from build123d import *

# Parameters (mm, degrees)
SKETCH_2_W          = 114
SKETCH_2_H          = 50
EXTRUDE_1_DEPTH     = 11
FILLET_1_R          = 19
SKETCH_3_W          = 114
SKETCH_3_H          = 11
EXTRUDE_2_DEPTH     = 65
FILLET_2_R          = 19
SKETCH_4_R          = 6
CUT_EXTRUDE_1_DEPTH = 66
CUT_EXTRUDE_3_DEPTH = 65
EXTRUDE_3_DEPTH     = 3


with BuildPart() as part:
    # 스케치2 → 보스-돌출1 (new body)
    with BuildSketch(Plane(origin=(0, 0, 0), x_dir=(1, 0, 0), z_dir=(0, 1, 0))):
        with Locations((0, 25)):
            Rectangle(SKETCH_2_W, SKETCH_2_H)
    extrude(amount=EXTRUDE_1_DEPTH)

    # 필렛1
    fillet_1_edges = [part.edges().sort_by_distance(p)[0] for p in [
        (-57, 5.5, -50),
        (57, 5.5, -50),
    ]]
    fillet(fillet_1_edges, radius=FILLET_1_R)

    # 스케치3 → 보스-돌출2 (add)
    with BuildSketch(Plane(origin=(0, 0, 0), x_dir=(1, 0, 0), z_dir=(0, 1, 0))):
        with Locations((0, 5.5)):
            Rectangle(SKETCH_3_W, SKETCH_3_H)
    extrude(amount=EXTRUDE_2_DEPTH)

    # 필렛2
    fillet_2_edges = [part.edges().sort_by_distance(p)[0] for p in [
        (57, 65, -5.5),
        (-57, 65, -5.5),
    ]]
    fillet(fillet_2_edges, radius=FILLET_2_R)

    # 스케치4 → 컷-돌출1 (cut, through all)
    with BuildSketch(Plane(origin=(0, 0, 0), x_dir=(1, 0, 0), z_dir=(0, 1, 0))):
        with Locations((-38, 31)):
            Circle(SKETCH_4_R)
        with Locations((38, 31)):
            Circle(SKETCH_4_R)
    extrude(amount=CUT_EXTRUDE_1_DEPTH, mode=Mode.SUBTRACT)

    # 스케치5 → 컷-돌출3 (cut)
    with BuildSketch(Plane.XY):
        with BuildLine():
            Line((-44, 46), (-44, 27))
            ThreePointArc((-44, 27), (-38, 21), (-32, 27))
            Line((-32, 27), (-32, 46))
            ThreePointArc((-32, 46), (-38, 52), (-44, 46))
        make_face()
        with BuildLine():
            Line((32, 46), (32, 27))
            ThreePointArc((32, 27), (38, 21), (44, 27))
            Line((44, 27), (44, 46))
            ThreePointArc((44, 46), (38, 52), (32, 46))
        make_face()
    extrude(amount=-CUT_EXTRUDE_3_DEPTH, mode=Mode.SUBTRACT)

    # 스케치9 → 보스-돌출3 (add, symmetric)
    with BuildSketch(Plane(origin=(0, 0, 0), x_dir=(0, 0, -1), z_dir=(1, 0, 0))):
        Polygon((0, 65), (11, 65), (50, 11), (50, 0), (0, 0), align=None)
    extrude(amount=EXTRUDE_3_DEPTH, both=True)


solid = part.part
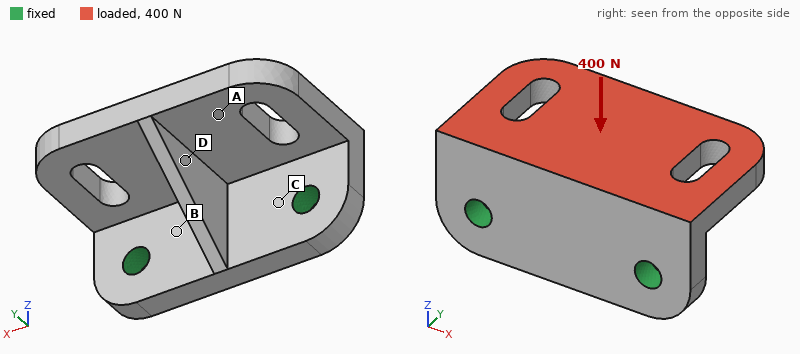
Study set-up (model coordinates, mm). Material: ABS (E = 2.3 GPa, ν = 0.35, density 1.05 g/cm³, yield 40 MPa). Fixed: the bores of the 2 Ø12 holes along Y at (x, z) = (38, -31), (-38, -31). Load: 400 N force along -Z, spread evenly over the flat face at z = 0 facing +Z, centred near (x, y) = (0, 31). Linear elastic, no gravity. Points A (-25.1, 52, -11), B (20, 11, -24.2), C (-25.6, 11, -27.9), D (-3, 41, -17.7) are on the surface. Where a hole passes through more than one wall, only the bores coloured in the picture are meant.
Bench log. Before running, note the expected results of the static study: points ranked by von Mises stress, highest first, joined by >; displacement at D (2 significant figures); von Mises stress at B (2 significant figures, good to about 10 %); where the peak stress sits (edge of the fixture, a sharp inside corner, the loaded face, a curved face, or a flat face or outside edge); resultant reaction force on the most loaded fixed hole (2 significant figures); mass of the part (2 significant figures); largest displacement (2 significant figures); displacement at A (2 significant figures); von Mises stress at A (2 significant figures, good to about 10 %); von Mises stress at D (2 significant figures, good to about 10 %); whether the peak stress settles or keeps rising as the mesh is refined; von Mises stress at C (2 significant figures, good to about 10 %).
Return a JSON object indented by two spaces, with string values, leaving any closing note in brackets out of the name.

{
  "points ranked by von Mises stress, highest first, joined by >": "C > B > D > A",
  "displacement at D": "0.23 mm",
  "von Mises stress at B": "2.4 MPa",
  "where the peak stress sits": "edge of the fixture",
  "resultant reaction force on the most loaded fixed hole": "200 N",
  "mass of the part": "130 g",
  "largest displacement": "0.46 mm",
  "displacement at A": "0.33 mm",
  "von Mises stress at A": "0.70 MPa",
  "von Mises stress at D": "1.5 MPa",
  "whether the peak stress settles or keeps rising as the mesh is refined": "keeps rising",
  "von Mises stress at C": "3.0 MPa"
}
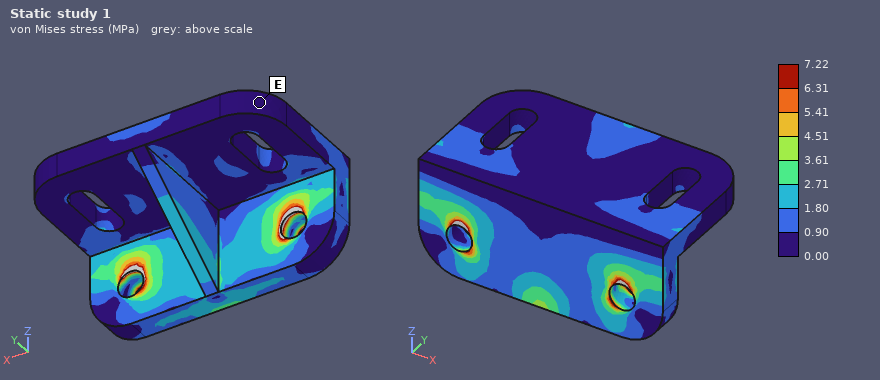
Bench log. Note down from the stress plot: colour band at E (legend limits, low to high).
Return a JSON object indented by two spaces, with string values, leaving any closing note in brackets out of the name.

{
  "colour band at E": "0.00 to 0.90 MPa"
}
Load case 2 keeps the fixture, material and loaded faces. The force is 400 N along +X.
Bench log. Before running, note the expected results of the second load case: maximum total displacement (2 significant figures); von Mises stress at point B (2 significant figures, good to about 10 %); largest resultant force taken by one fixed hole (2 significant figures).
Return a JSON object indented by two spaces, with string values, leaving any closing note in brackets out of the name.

{
  "maximum total displacement": "80 µm",
  "von Mises stress at point B": "1.1 MPa",
  "largest resultant force taken by one fixed hole": "280 N"
}
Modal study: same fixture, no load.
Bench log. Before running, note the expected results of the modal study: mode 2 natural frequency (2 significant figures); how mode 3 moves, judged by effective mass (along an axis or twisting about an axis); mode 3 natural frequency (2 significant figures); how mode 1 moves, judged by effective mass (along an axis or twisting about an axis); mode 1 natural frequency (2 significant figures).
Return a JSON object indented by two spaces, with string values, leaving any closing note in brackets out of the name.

{
  "mode 2 natural frequency": "940 Hz",
  "how mode 3 moves, judged by effective mass": "along X",
  "mode 3 natural frequency": "1400 Hz",
  "how mode 1 moves, judged by effective mass": "along Z",
  "mode 1 natural frequency": "610 Hz"
}
